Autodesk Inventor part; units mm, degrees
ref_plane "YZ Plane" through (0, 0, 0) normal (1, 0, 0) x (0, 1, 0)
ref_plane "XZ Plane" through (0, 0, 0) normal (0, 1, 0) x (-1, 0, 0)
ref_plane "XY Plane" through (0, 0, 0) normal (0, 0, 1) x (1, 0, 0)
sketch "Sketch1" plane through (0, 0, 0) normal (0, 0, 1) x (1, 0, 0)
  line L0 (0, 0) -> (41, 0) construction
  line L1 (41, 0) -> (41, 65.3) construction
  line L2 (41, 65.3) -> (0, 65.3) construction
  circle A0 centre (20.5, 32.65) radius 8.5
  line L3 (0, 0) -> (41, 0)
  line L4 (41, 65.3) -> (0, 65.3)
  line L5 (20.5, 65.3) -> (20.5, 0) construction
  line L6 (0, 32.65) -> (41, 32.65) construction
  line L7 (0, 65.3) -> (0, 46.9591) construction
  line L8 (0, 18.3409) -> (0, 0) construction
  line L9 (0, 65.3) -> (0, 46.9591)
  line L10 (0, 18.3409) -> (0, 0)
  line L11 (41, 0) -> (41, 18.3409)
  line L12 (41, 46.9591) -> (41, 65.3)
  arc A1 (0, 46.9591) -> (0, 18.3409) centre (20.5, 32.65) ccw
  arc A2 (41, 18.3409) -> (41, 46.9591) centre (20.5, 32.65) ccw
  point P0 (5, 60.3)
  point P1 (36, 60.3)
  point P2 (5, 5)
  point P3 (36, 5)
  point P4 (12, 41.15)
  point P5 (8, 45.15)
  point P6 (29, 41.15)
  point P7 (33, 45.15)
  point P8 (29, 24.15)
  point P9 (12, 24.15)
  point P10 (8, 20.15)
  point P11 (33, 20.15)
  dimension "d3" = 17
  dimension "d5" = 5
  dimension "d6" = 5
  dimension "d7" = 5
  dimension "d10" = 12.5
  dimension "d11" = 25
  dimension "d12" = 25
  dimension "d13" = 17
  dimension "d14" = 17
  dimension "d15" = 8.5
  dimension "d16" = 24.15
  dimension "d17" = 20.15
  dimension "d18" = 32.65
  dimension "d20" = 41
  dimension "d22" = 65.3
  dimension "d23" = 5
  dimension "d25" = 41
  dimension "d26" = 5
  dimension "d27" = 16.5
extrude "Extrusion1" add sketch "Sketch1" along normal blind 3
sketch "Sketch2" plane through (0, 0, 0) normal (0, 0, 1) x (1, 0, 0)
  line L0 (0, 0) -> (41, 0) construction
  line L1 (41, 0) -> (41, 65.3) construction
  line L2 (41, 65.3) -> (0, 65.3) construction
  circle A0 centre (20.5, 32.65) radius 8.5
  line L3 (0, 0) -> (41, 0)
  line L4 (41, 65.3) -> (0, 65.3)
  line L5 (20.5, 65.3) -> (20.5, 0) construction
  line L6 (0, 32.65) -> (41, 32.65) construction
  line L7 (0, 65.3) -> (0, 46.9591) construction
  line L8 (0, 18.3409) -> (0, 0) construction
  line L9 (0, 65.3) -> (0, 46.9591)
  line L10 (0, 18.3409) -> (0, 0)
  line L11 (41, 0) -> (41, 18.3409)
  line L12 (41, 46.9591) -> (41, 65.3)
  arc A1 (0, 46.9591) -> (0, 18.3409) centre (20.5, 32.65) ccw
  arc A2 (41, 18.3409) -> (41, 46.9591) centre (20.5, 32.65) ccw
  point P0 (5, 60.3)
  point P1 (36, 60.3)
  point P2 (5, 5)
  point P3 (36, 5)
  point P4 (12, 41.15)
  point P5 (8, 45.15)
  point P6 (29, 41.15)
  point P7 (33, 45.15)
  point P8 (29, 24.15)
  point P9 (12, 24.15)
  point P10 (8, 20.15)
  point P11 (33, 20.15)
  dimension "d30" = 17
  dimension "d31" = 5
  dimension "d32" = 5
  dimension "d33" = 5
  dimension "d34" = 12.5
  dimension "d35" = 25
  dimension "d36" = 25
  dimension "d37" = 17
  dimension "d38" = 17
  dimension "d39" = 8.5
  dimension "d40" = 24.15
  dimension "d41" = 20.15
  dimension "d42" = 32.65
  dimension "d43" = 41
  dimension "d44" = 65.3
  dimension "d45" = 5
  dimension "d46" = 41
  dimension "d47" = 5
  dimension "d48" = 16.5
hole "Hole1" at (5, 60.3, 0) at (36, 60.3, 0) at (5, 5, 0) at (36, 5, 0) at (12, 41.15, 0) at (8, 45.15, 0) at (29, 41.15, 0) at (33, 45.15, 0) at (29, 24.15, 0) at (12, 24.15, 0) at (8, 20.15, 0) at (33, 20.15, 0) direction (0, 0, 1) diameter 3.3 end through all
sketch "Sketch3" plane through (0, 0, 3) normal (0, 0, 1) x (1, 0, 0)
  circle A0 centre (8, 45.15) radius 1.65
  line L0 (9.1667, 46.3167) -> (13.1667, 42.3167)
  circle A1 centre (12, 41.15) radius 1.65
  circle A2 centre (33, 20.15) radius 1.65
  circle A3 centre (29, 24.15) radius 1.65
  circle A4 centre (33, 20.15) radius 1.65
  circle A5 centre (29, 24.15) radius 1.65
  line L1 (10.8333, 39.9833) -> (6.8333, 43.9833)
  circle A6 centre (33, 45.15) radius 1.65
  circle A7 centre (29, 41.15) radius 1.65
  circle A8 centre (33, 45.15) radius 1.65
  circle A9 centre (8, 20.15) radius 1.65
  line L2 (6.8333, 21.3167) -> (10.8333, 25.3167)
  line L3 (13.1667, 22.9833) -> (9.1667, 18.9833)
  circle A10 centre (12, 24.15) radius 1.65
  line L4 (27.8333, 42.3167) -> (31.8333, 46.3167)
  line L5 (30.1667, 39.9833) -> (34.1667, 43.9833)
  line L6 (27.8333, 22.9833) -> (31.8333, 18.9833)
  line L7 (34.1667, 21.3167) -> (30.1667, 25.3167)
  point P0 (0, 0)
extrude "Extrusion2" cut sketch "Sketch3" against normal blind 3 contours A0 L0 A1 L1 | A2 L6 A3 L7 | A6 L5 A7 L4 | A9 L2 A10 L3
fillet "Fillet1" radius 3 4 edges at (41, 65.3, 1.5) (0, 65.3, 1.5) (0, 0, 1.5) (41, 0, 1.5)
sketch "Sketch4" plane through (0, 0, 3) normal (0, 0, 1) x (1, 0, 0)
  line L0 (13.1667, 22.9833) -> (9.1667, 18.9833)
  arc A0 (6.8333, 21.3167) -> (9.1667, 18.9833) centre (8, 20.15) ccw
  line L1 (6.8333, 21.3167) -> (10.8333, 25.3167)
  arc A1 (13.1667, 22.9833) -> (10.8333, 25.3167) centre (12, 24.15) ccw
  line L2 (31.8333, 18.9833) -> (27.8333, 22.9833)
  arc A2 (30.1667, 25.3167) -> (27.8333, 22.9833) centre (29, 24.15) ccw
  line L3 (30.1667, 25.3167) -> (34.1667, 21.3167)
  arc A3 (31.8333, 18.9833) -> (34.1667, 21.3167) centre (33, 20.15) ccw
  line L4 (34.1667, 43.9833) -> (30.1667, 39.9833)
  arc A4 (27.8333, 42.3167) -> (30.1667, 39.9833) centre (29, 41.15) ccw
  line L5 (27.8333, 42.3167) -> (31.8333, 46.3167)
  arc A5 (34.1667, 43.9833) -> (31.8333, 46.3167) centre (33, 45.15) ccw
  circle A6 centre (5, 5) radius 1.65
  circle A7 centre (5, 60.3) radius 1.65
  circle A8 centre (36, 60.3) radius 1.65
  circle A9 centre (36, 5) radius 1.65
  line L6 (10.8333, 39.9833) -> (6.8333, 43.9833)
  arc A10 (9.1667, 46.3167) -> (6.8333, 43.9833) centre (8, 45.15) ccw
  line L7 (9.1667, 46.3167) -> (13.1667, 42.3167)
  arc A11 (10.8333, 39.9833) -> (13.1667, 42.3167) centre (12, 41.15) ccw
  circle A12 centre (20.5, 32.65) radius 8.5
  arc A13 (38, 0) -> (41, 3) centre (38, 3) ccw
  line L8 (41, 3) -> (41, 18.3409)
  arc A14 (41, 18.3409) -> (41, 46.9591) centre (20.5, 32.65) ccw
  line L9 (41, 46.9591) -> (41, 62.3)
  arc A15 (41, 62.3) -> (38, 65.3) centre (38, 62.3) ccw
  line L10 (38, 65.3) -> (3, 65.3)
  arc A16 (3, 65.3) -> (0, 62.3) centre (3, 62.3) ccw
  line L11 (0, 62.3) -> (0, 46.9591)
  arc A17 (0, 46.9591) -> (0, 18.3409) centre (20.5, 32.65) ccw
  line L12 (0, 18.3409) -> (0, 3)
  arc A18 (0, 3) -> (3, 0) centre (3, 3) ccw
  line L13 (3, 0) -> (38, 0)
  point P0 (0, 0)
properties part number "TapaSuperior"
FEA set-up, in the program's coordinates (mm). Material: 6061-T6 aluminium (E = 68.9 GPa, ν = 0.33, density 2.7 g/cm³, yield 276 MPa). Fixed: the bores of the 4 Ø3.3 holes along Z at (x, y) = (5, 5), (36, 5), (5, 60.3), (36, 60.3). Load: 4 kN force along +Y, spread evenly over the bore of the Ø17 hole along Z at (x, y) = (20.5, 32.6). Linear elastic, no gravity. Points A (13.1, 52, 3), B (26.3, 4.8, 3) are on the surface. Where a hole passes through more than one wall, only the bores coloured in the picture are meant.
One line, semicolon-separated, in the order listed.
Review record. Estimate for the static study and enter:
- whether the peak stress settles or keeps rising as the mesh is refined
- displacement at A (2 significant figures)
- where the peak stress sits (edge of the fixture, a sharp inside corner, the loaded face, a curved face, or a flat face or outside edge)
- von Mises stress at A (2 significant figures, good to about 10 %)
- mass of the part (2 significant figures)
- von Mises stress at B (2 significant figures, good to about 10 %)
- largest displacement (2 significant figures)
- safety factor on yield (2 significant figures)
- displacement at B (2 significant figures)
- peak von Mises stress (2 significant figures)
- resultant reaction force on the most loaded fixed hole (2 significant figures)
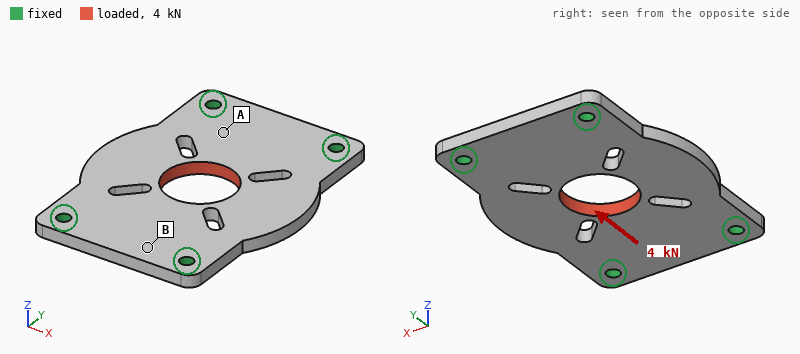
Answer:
settles; 5.5 µm; a curved face; 25 MPa; 20 g; 9.7 MPa; 13 µm; 2.5; 5.1 µm; 110 MPa; 1.0 kN
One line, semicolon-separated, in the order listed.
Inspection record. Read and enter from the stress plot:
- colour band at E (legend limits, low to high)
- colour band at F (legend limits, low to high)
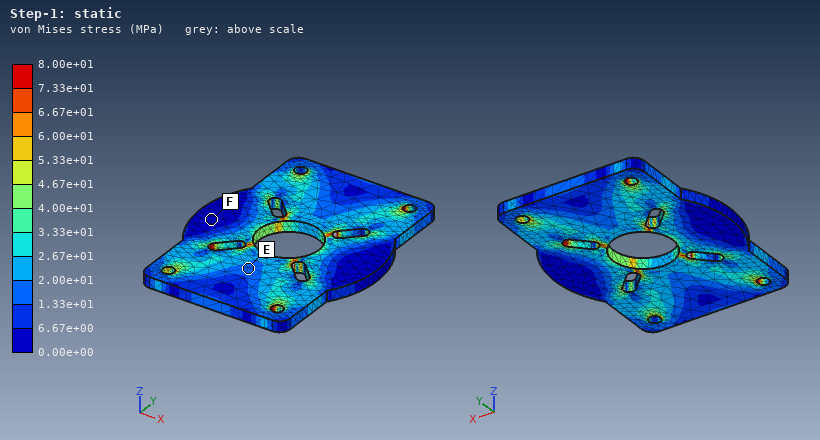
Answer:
1.33e+01 to 2.00e+01 MPa; 0.00e+00 to 6.67e+00 MPa
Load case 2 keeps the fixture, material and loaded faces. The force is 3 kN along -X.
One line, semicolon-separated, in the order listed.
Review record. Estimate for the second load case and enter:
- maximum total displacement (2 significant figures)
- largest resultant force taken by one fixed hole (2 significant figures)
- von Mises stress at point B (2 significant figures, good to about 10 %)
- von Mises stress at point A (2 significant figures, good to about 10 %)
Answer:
18 µm; 900 N; 12 MPa; 27 MPa
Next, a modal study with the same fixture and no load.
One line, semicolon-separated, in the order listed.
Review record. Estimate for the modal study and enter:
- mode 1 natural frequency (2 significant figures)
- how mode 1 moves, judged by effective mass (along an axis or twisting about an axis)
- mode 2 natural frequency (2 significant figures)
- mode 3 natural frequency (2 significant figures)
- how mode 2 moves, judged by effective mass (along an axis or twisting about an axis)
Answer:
4600 Hz; along Z; 5600 Hz; 8600 Hz; twisting about Y
